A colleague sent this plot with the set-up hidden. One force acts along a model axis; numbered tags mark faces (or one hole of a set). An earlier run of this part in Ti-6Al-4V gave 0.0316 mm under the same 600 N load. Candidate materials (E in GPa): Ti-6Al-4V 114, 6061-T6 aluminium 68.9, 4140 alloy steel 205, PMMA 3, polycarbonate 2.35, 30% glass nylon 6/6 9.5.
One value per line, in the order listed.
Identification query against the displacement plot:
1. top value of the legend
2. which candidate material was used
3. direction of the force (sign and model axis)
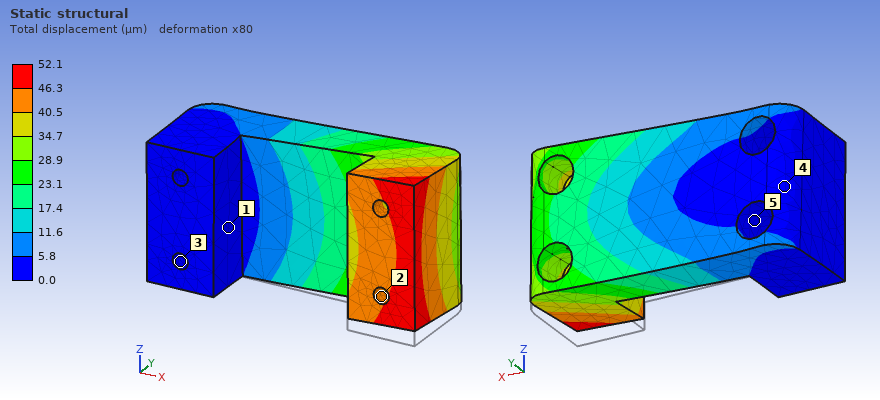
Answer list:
52.1 µm
6061-T6 aluminium
+Z
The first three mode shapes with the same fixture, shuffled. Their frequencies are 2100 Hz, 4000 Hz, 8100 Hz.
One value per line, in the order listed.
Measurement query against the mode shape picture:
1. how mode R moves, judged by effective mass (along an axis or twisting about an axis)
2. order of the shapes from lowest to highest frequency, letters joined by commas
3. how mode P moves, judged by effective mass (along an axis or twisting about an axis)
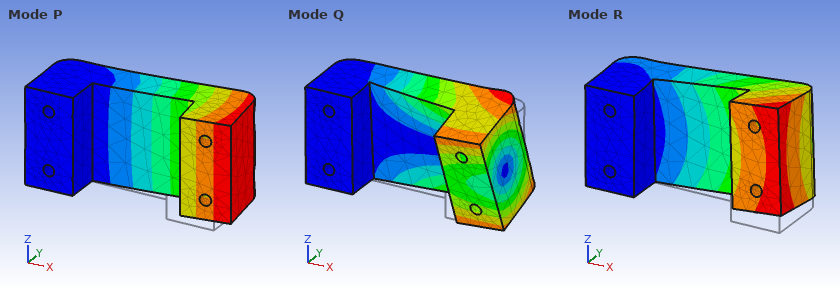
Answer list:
along Z
P, R, Q
along Y
